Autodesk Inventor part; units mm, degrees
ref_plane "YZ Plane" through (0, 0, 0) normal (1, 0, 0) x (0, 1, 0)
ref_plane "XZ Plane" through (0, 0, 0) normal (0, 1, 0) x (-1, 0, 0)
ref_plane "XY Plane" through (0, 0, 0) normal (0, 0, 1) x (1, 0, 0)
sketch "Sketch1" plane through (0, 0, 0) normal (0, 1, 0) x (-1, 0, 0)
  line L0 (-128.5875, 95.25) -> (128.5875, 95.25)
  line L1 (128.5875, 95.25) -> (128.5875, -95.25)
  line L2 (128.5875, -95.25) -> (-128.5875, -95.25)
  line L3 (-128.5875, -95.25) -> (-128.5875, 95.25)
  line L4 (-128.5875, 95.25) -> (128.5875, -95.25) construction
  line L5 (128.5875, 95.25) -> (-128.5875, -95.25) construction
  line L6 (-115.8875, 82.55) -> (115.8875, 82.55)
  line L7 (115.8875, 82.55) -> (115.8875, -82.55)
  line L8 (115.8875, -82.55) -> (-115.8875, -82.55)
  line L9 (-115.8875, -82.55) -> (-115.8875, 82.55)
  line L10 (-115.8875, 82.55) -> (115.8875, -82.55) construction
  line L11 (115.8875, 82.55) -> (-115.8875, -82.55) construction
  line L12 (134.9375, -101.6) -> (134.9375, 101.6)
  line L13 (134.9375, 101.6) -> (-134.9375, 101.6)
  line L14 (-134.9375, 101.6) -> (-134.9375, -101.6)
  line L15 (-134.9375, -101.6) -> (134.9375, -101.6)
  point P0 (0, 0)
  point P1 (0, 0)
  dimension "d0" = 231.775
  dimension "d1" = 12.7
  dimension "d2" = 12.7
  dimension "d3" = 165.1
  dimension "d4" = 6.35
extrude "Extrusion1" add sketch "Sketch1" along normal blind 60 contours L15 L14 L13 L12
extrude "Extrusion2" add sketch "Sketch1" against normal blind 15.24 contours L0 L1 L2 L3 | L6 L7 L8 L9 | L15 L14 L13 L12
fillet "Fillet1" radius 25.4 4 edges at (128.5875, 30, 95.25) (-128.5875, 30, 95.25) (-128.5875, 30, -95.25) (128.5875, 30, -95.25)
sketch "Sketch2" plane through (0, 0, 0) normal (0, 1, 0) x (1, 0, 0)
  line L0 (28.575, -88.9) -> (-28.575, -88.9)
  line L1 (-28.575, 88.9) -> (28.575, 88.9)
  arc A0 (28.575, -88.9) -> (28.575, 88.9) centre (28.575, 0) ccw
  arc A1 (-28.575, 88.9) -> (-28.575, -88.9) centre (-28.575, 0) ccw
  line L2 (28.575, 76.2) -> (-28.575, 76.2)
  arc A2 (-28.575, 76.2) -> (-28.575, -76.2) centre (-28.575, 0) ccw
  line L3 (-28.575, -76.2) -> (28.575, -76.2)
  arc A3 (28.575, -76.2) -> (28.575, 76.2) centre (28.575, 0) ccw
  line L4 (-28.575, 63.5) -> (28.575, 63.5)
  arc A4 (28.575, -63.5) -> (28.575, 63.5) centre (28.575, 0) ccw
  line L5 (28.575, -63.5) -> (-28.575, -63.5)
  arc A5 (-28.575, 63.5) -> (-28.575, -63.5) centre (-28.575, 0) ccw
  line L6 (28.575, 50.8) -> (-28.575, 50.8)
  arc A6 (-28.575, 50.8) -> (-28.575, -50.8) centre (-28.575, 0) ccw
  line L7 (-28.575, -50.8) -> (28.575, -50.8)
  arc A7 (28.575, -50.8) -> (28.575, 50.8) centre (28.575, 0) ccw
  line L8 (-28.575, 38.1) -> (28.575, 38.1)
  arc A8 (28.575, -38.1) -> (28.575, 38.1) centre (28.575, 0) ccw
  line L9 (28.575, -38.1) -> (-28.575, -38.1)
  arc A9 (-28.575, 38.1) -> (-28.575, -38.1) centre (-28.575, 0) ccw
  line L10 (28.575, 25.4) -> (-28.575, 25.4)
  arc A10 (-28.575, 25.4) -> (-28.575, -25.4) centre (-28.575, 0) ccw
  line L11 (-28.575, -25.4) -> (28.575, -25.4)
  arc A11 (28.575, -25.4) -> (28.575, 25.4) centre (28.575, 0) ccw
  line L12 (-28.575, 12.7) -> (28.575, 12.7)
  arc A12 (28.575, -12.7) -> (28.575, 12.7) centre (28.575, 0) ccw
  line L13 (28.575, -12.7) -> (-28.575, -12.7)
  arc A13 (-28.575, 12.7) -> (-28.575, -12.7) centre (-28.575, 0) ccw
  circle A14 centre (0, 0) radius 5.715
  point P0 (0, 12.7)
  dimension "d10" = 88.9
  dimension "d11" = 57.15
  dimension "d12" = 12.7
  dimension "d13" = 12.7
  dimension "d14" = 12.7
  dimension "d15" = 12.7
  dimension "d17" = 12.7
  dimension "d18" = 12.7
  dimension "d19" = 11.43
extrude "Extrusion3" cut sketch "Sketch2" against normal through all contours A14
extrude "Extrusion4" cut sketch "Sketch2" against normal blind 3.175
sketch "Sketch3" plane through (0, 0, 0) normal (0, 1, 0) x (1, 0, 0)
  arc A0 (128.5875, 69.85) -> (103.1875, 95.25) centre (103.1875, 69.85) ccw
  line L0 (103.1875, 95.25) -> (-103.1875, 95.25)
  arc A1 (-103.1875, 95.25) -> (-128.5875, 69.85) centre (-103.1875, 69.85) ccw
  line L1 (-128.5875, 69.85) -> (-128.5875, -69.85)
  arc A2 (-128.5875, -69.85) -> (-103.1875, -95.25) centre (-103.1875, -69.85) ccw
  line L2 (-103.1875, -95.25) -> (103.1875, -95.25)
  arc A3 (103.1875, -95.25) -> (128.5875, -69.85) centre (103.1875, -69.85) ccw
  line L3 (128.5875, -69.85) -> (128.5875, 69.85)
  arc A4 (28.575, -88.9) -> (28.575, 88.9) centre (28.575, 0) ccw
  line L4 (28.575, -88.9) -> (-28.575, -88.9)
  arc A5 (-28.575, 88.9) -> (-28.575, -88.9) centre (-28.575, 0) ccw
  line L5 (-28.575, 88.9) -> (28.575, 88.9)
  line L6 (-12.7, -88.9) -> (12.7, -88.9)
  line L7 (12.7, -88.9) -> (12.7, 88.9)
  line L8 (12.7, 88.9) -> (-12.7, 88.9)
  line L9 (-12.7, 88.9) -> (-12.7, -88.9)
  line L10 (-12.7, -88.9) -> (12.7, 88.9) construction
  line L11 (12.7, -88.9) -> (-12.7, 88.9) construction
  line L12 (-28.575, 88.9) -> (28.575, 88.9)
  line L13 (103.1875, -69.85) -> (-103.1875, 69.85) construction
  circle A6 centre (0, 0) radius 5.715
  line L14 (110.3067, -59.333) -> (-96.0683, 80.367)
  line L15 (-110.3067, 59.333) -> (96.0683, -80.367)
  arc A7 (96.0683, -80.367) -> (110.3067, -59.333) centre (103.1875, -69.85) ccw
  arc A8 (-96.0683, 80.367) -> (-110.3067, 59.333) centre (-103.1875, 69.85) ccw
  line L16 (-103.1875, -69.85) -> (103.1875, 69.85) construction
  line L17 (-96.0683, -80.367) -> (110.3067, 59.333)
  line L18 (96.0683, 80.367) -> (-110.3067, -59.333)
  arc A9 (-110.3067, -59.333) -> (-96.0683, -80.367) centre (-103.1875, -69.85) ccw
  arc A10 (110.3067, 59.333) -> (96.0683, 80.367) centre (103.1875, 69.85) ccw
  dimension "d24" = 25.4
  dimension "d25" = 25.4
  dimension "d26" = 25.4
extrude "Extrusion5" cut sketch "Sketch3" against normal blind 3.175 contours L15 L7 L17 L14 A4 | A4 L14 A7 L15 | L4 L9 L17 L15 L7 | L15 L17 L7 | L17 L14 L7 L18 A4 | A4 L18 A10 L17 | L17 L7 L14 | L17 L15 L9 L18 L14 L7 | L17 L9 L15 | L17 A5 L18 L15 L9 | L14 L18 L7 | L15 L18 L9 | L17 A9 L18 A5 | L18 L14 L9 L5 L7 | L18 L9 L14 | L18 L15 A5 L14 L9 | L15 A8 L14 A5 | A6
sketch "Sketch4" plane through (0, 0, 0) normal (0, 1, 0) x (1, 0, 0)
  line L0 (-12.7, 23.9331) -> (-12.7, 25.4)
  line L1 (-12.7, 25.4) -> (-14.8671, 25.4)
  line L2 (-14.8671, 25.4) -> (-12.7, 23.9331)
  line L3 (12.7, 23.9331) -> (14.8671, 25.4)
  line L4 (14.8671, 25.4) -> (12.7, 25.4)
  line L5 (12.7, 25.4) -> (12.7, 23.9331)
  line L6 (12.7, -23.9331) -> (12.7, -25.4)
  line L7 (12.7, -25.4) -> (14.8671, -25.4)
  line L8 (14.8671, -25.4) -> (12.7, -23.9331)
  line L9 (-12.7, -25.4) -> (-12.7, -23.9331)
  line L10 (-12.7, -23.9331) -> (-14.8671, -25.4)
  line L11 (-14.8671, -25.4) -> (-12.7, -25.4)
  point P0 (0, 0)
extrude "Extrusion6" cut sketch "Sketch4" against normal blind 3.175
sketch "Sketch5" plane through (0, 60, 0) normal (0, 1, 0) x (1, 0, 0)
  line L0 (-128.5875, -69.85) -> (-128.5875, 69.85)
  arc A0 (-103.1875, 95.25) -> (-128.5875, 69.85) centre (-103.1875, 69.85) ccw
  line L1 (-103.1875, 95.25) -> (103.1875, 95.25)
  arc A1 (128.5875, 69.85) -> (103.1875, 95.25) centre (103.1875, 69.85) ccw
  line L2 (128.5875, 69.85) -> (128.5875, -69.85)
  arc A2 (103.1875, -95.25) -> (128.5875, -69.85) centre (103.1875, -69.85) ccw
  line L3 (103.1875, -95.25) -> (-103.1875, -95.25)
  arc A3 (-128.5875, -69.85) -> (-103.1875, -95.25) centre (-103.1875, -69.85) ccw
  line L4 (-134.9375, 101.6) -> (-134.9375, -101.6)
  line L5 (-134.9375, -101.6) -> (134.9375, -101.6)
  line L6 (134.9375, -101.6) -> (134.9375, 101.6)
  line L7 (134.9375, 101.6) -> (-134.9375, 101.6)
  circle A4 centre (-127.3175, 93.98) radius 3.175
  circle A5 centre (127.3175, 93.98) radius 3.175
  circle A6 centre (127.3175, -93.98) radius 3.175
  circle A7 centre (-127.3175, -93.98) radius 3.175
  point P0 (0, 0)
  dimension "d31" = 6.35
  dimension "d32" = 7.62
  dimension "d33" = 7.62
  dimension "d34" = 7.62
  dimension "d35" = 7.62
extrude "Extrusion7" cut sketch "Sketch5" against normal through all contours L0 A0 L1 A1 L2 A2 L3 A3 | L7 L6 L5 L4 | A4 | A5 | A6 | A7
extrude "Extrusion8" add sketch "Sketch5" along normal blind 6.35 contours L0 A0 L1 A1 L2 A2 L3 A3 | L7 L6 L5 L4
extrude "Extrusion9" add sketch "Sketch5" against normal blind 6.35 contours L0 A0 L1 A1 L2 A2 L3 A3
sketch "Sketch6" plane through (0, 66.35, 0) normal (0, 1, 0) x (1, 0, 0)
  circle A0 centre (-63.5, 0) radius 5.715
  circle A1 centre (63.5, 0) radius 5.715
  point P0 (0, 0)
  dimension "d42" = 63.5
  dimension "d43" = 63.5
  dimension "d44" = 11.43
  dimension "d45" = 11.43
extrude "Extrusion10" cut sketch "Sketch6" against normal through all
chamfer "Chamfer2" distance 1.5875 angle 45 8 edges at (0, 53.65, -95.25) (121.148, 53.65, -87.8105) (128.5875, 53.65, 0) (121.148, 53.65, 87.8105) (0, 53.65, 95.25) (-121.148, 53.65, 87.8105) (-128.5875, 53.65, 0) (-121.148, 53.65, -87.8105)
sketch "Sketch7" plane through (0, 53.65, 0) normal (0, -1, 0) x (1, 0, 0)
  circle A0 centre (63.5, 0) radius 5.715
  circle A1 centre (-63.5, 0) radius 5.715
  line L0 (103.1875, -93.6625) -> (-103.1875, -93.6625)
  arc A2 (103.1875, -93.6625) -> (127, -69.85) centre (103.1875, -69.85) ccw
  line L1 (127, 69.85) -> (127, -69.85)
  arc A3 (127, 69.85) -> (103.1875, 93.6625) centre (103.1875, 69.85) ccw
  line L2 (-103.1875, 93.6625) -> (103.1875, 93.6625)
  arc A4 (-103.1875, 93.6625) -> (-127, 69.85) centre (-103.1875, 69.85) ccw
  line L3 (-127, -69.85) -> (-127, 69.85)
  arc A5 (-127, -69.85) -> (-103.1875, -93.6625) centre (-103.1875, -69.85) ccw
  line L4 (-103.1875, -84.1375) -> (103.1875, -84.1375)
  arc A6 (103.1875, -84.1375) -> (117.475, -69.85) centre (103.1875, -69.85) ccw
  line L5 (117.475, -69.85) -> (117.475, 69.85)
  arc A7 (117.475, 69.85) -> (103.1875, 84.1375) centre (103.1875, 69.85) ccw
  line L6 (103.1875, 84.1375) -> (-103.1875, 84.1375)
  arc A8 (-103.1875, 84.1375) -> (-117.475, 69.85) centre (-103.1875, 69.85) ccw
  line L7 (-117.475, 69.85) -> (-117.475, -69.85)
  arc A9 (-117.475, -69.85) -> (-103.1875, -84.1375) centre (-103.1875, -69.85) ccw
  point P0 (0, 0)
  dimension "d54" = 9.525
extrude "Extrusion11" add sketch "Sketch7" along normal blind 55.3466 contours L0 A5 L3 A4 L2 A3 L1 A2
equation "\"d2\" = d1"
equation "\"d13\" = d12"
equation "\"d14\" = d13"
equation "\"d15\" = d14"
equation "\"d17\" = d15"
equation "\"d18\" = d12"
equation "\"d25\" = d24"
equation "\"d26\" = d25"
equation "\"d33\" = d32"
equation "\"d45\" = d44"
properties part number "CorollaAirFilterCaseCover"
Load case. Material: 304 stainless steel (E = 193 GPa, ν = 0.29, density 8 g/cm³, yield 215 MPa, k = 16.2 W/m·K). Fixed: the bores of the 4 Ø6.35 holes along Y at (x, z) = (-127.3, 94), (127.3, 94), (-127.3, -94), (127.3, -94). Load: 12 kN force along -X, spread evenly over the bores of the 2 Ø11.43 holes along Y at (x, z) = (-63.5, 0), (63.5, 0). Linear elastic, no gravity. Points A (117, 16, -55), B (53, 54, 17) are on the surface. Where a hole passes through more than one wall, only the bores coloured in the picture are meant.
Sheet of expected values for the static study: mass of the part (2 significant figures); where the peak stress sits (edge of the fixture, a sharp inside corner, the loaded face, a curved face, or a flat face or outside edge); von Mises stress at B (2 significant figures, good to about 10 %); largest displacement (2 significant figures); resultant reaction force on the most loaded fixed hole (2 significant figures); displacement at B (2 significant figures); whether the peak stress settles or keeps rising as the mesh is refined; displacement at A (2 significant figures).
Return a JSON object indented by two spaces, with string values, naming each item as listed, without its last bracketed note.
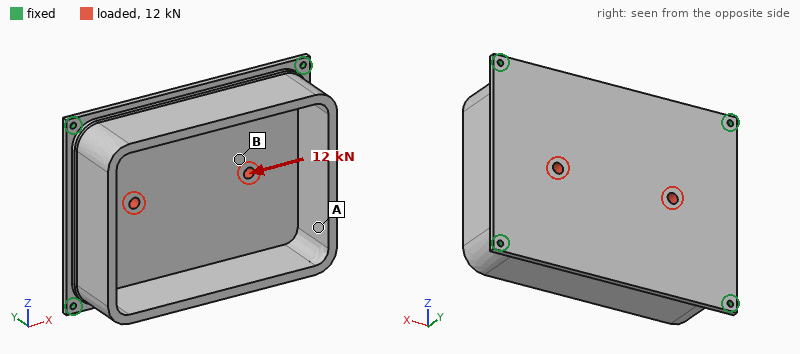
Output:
{
  "mass of the part": "8.6 kg",
  "where the peak stress sits": "edge of the fixture",
  "von Mises stress at B": "5.4 MPa",
  "largest displacement": "6.6 µm",
  "resultant reaction force on the most loaded fixed hole": "3.3 kN",
  "displacement at B": "5.4 µm",
  "whether the peak stress settles or keeps rising as the mesh is refined": "keeps rising",
  "displacement at A": "4.5 µm"
}
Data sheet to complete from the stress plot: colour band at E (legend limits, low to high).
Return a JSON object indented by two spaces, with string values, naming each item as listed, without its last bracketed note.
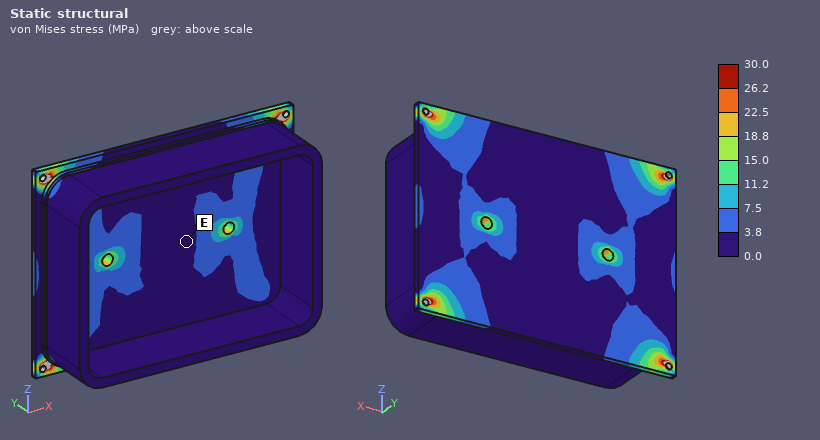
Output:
{
  "colour band at E": "0.0 to 3.8 MPa"
}
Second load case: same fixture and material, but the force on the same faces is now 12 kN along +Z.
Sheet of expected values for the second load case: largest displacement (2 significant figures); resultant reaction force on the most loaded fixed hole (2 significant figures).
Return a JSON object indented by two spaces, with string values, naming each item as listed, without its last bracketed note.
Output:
{
  "largest displacement": "6.4 µm",
  "resultant reaction force on the most loaded fixed hole": "3.3 kN"
}
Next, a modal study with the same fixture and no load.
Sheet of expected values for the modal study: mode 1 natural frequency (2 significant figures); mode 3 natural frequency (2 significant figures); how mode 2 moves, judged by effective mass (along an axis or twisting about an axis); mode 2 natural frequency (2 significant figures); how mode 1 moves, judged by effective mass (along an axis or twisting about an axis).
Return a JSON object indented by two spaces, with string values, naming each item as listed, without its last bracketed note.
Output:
{
  "mode 1 natural frequency": "1200 Hz",
  "mode 3 natural frequency": "1900 Hz",
  "how mode 2 moves, judged by effective mass": "along Z",
  "mode 2 natural frequency": "1800 Hz",
  "how mode 1 moves, judged by effective mass": "along Y"
}
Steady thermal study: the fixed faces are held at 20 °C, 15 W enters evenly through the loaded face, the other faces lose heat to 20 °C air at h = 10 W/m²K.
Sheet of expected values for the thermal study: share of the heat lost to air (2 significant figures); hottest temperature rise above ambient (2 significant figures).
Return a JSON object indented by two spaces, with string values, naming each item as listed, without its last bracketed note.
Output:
{
  "share of the heat lost to air": "81 %",
  "hottest temperature rise above ambient": "20 K"
}
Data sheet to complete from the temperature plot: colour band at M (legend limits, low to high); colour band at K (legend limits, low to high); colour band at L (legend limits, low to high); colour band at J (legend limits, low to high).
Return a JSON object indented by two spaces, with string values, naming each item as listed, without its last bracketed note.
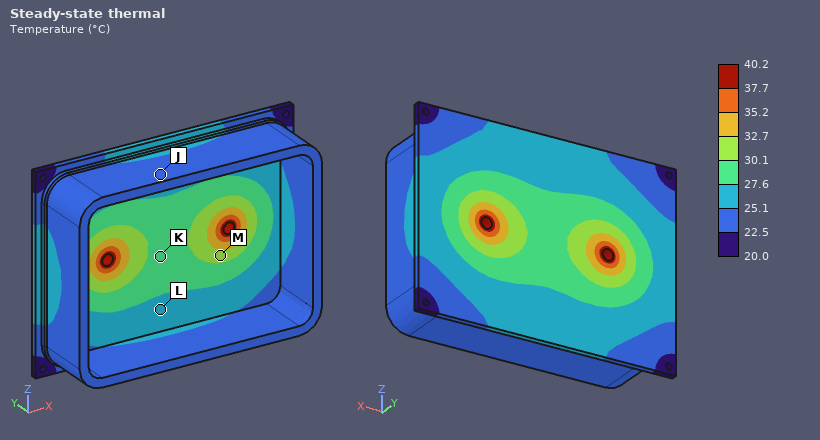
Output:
{
  "colour band at M": "30.1 to 32.7 °C",
  "colour band at K": "27.6 to 30.1 °C",
  "colour band at L": "25.1 to 27.6 °C",
  "colour band at J": "22.5 to 25.1 °C"
}
